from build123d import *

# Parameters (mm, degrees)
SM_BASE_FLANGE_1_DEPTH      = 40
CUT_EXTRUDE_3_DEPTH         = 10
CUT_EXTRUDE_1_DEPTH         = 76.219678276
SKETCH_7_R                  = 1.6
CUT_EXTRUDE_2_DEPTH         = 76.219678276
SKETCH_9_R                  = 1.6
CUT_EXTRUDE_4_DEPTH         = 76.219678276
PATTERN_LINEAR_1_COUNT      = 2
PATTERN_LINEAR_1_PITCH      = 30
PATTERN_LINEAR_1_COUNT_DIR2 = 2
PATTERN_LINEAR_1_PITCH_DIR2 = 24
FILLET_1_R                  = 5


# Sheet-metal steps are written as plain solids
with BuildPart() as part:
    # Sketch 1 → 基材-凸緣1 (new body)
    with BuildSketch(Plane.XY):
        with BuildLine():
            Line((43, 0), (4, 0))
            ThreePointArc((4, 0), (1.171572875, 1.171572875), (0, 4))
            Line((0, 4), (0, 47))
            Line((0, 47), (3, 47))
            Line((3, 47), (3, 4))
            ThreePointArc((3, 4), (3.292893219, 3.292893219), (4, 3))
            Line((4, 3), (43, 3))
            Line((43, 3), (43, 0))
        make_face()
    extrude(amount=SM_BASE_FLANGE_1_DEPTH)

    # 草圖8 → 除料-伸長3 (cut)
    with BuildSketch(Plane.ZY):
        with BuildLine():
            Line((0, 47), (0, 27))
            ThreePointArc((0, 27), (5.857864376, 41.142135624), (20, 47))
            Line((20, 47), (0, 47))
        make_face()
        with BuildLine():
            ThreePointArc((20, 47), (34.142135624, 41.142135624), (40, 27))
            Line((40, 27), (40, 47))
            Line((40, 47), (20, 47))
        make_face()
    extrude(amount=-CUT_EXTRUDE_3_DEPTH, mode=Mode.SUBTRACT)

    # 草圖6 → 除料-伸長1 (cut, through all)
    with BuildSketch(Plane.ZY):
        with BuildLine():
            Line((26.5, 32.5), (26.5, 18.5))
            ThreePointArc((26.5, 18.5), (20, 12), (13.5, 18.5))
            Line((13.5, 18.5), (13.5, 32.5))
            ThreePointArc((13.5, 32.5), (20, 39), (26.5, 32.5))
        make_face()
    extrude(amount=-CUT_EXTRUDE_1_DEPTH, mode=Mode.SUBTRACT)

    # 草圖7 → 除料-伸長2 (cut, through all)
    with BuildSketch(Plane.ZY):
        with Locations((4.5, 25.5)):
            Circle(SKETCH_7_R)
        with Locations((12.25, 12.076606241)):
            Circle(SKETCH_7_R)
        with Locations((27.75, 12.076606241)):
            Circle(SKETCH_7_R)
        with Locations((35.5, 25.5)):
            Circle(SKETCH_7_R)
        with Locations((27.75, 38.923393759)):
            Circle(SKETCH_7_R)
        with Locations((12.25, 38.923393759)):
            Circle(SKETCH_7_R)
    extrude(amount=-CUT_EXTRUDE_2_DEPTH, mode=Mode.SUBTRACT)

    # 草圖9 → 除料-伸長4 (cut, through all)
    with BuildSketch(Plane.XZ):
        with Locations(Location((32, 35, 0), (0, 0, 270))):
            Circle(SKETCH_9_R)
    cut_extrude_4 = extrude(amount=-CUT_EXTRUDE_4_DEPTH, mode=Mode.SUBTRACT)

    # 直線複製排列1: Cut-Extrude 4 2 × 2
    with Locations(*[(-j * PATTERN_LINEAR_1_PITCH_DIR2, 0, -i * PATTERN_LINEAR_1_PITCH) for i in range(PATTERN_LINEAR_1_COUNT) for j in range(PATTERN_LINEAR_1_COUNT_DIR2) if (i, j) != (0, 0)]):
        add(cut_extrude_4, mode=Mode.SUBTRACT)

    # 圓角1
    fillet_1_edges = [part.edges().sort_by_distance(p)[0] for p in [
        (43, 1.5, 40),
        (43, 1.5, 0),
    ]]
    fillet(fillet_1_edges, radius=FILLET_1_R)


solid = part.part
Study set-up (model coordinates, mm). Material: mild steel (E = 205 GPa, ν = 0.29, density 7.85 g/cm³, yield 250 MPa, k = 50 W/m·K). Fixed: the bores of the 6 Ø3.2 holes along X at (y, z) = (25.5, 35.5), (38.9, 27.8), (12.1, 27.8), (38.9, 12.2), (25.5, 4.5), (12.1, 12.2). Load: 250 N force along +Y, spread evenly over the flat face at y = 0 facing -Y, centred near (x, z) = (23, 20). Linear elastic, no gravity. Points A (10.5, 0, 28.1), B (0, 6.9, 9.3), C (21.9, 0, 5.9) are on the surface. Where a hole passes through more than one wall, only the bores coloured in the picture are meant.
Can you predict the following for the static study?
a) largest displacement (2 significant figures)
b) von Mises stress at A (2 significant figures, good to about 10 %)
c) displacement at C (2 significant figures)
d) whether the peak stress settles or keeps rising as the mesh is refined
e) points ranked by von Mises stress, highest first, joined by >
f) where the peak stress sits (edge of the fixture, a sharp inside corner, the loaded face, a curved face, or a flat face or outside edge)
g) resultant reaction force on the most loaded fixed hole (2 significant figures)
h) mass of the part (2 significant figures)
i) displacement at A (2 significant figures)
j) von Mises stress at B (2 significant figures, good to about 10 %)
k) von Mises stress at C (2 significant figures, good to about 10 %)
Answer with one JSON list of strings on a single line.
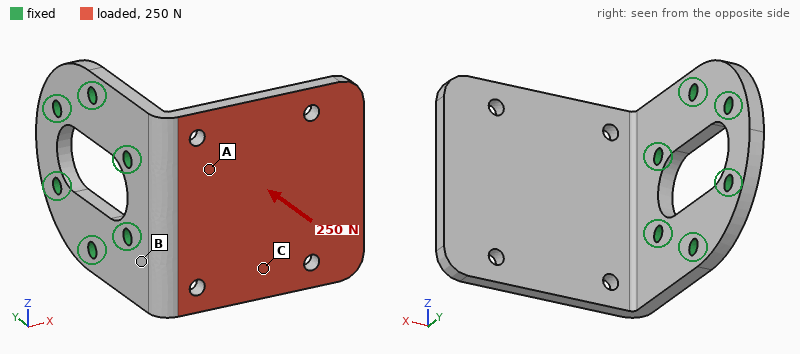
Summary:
["0.25 mm", "55 MPa", "0.11 mm", "keeps rising", "B > A > C", "edge of the fixture", "130 N", "67 g", "0.045 mm", "86 MPa", "23 MPa"]
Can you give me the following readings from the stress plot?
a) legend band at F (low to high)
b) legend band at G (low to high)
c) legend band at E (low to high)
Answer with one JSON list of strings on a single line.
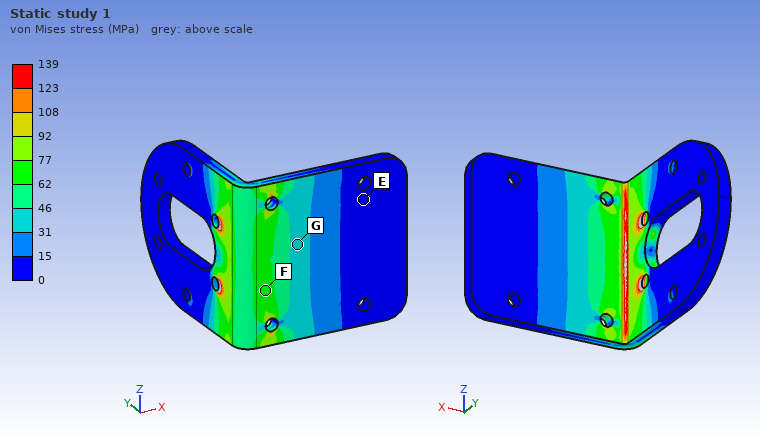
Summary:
["62 to 77 MPa", "31 to 46 MPa", "0 to 15 MPa"]
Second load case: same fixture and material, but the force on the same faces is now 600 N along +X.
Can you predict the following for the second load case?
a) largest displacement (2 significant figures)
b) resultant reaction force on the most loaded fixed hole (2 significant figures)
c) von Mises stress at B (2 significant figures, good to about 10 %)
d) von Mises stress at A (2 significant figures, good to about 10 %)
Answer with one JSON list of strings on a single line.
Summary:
["0.13 mm", "360 N", "71 MPa", "18 MPa"]
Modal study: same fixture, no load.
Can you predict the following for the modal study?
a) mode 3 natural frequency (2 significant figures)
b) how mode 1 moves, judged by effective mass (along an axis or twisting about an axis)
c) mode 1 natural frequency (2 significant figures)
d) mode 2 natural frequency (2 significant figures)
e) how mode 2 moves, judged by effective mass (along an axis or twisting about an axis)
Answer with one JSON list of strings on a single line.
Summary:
["3700 Hz", "along Y", "1000 Hz", "2500 Hz", "along Z"]
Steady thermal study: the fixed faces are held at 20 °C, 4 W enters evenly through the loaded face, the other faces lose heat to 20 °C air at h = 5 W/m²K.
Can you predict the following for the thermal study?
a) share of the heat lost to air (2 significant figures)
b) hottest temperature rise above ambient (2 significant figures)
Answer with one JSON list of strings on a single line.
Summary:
["5.1 %", "22 K"]
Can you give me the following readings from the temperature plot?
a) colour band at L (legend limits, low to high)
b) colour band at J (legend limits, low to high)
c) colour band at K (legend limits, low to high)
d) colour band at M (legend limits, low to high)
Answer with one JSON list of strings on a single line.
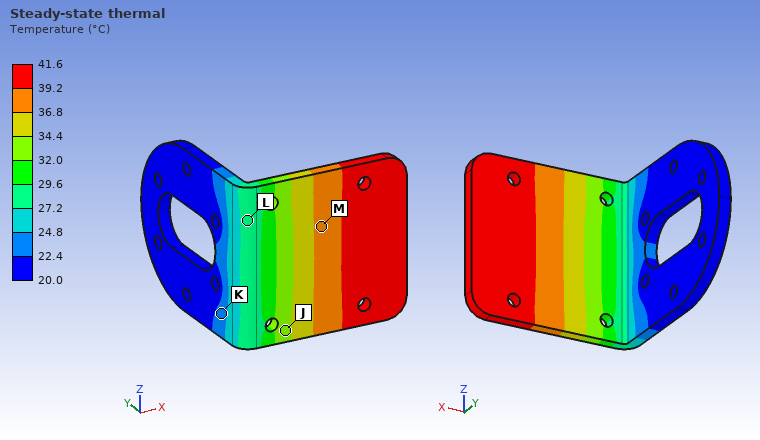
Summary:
["27.2 to 29.6 °C", "32.0 to 34.4 °C", "22.4 to 24.8 °C", "36.8 to 39.2 °C"]
